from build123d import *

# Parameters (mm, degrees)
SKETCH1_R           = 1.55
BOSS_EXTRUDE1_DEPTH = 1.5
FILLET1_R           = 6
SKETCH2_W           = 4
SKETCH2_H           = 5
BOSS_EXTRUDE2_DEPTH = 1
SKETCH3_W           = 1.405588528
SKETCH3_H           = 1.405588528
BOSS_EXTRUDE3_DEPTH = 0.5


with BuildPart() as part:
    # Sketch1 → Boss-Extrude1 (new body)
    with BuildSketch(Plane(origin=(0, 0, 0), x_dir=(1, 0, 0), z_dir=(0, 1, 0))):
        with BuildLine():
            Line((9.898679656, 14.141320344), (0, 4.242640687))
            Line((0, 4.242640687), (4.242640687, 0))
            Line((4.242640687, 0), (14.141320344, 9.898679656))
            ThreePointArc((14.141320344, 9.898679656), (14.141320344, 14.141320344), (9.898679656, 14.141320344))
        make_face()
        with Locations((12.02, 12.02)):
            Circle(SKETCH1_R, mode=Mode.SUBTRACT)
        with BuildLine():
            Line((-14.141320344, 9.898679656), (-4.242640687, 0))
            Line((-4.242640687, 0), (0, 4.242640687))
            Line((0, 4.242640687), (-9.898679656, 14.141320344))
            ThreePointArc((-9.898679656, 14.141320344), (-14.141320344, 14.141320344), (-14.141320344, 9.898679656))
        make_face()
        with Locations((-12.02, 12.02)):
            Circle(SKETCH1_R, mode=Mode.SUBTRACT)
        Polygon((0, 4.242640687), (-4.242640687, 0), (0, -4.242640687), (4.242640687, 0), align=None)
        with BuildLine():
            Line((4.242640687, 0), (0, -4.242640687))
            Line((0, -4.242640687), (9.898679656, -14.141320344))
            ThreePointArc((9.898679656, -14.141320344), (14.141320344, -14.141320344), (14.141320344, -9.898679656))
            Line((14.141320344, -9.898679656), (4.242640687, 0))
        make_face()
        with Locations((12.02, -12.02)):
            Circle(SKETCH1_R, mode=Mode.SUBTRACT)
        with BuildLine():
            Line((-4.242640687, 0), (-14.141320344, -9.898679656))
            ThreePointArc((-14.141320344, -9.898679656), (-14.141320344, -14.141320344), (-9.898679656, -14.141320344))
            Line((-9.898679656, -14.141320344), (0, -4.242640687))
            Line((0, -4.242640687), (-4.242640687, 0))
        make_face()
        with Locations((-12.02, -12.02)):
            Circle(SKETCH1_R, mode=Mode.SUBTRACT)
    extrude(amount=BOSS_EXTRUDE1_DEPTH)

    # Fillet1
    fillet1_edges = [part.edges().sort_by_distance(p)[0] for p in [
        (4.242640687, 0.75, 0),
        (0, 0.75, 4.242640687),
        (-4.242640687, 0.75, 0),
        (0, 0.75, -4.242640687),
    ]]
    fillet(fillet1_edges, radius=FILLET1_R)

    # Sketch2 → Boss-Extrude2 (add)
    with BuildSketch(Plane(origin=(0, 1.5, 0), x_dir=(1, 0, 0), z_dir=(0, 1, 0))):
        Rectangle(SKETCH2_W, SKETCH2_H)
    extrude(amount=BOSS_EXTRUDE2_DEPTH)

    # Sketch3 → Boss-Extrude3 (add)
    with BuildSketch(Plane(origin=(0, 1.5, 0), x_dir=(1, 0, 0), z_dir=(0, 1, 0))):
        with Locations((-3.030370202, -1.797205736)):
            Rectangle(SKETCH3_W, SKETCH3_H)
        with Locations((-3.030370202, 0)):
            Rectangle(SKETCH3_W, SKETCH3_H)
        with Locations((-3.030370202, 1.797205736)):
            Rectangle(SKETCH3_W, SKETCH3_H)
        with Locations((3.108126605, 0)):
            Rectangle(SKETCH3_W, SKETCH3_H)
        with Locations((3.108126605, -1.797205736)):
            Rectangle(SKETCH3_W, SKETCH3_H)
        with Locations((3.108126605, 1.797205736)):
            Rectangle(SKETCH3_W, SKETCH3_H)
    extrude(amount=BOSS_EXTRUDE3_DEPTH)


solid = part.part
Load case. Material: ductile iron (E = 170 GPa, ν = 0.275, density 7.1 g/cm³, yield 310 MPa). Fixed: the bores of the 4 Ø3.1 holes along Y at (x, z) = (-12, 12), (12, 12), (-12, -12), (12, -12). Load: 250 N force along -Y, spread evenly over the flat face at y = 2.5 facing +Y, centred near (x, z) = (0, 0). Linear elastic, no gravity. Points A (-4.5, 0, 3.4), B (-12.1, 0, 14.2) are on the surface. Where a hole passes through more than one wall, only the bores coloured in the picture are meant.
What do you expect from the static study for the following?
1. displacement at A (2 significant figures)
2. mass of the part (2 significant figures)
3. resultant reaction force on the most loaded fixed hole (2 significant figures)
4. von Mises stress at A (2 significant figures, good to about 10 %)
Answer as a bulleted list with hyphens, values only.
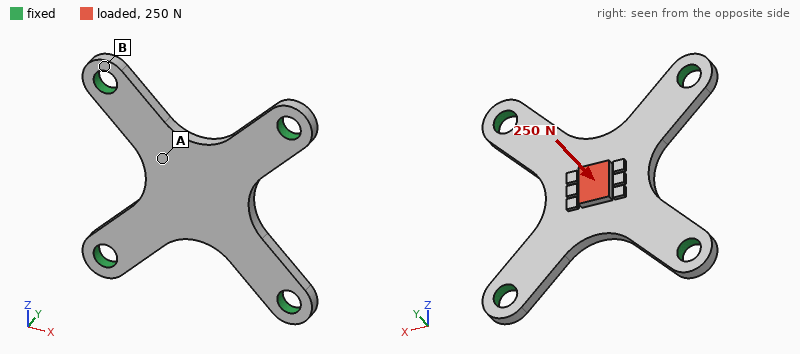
- 34 µm
- 4.8 g
- 64 N
- 69 MPa
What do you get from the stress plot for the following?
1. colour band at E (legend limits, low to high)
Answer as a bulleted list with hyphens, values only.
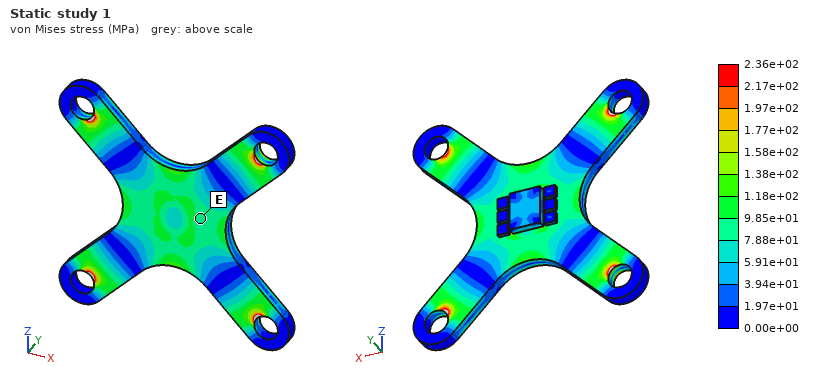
- 7.88e+01 to 9.85e+01 MPa
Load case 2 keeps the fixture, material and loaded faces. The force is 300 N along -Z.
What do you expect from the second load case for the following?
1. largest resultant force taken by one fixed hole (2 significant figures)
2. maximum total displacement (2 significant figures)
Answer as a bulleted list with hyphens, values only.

- 97 N
- 6.8 µm
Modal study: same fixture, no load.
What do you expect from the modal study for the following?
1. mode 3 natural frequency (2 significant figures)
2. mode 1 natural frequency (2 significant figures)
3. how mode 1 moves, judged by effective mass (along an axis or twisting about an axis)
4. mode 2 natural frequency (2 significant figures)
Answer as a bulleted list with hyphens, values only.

- 20 kHz
- 9000 Hz
- along Y
- 20 kHz
